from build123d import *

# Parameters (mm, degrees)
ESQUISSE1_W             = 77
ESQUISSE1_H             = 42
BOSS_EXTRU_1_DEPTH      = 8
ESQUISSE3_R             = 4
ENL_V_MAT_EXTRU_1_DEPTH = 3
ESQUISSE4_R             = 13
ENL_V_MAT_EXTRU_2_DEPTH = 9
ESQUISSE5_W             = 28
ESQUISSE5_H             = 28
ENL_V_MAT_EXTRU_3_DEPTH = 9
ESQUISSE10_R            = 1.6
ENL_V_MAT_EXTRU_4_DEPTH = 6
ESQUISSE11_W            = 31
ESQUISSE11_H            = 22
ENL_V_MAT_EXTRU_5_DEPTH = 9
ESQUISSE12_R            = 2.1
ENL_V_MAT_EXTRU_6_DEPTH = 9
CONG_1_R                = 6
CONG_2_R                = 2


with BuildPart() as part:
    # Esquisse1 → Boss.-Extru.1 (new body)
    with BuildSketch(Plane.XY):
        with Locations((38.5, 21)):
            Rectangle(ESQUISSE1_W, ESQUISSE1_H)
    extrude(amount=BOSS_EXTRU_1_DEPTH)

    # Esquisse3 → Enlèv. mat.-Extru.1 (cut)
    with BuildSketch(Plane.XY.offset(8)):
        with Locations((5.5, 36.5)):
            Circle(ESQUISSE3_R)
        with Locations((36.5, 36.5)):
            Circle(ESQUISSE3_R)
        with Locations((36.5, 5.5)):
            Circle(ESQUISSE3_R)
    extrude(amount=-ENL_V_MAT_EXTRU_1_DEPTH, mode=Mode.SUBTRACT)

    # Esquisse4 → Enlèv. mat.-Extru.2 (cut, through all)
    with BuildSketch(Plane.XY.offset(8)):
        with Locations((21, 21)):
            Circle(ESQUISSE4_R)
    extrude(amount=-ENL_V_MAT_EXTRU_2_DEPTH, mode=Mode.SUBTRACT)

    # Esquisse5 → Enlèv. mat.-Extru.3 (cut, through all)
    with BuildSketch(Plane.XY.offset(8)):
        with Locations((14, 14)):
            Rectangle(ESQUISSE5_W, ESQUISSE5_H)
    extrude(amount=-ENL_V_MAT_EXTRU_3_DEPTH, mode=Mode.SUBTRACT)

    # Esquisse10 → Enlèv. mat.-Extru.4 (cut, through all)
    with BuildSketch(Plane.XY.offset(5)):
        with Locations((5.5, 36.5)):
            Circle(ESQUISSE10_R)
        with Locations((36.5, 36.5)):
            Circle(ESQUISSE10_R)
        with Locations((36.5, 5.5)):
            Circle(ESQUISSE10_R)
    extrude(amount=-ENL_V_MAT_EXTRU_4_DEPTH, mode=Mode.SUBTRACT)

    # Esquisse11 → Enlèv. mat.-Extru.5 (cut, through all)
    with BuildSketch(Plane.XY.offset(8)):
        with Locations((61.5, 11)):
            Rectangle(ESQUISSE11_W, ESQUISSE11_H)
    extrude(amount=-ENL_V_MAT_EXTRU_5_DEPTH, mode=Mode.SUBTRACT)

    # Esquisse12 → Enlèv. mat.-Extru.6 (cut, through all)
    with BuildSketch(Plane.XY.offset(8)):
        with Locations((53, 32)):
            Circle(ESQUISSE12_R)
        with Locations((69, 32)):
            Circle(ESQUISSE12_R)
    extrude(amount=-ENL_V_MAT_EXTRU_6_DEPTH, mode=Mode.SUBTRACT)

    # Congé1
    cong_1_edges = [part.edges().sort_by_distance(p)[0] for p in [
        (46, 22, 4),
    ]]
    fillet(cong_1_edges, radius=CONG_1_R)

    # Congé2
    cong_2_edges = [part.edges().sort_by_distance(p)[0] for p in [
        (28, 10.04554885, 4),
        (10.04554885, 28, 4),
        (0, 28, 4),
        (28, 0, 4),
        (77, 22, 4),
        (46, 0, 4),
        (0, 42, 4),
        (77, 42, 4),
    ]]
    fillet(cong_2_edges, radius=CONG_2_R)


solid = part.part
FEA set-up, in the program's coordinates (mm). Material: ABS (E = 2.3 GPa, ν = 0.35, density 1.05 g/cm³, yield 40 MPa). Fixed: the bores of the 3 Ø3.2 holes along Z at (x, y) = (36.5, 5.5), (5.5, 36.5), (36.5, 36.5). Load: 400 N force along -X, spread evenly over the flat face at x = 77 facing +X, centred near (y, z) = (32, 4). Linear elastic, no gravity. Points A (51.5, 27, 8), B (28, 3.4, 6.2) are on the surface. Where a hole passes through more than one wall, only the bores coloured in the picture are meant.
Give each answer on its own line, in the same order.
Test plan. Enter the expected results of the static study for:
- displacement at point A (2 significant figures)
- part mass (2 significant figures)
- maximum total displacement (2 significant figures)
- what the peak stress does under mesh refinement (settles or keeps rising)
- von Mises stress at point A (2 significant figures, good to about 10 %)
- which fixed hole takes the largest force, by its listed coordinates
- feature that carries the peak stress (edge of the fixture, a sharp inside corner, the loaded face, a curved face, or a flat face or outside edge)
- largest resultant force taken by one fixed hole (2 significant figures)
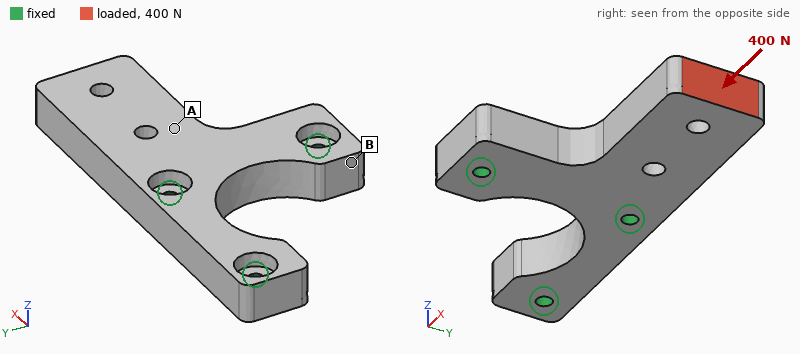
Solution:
0.057 mm
13 g
0.13 mm
keeps rising
2.6 MPa
(36.5, 36.5)
edge of the fixture
320 N
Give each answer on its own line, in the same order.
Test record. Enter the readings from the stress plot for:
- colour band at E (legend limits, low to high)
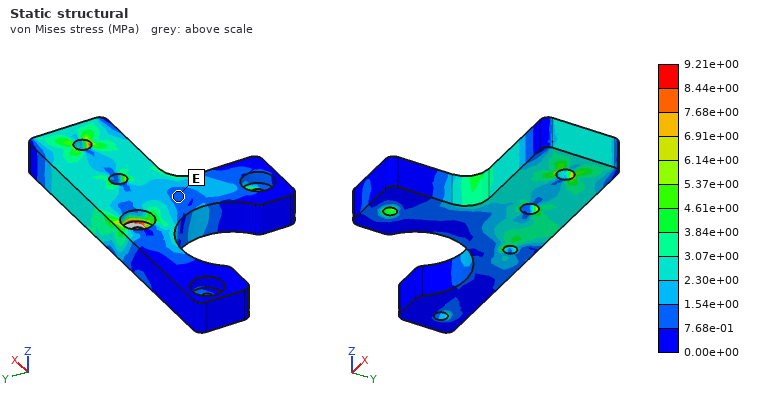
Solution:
7.68e-01 to 1.54e+00 MPa
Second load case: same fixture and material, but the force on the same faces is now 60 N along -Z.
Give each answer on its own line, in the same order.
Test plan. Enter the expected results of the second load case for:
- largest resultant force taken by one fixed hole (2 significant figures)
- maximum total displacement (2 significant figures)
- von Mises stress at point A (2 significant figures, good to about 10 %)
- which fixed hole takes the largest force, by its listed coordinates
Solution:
89 N
1.0 mm
8.5 MPa
(36.5, 36.5)
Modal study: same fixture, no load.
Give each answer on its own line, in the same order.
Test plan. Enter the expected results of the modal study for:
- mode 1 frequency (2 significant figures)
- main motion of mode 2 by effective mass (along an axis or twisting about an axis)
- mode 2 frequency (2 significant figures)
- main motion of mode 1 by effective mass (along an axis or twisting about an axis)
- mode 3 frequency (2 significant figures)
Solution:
930 Hz
along Y
2500 Hz
along Z
3700 Hz
